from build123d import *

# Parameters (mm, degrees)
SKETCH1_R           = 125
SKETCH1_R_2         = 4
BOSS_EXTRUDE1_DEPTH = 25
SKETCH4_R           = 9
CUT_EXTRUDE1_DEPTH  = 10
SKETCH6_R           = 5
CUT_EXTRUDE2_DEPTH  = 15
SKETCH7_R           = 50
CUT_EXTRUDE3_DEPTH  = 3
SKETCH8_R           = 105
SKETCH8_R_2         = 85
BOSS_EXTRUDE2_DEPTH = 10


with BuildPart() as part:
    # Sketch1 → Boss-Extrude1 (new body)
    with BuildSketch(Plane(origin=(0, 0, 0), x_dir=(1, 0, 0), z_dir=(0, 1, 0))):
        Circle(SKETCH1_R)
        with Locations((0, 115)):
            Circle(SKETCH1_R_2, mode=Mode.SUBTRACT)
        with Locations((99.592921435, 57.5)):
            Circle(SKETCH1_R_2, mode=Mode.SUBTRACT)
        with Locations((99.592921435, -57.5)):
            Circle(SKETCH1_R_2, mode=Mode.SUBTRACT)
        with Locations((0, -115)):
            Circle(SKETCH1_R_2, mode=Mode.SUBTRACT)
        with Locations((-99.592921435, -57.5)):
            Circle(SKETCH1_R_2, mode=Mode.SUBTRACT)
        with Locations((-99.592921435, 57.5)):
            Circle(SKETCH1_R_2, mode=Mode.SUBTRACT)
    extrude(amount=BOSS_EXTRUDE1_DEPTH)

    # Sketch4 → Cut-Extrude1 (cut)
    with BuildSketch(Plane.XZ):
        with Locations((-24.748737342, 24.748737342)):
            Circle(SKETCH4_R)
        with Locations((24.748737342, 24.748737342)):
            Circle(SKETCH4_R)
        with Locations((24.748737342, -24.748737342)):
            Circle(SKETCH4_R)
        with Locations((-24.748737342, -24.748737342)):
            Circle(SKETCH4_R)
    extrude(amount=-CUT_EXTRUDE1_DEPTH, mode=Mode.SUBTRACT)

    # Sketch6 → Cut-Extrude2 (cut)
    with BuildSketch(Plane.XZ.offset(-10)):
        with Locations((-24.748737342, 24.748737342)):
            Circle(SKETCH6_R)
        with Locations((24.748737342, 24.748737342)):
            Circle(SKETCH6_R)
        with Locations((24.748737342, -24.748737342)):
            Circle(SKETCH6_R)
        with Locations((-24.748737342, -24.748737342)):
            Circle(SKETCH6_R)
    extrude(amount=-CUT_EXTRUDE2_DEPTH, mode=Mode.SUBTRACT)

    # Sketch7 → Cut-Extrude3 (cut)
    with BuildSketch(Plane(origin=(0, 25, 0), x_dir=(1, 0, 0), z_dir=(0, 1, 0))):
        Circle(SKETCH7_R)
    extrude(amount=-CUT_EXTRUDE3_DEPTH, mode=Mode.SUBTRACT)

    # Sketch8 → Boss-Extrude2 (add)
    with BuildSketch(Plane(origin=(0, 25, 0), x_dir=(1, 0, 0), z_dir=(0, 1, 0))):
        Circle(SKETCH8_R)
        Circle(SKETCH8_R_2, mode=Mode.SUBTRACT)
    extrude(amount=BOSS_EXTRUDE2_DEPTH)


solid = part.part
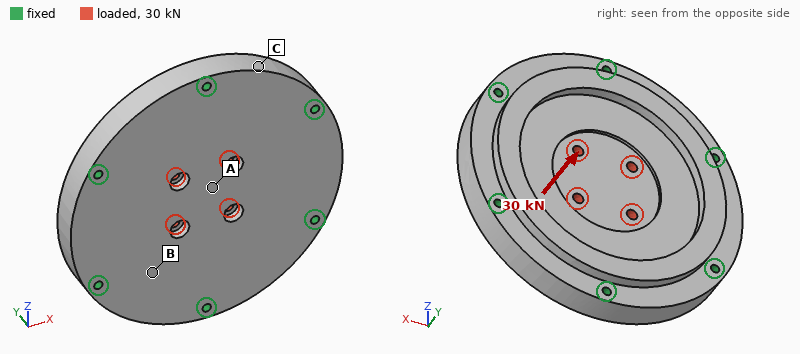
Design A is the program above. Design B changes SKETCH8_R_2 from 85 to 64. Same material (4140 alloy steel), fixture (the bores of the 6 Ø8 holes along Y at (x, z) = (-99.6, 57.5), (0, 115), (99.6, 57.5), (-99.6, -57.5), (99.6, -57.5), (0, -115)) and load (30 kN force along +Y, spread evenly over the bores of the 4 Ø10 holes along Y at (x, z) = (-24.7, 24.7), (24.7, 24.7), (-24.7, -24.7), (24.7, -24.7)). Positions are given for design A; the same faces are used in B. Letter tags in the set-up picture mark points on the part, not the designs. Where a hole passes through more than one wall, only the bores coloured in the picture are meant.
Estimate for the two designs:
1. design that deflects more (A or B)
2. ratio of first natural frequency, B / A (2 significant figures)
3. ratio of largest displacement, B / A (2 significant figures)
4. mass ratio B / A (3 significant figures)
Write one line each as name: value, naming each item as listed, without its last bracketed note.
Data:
design that deflects more: A
ratio of first natural frequency, B / A: 1.0
ratio of largest displacement, B / A: 0.85
mass ratio B / A: 1.08
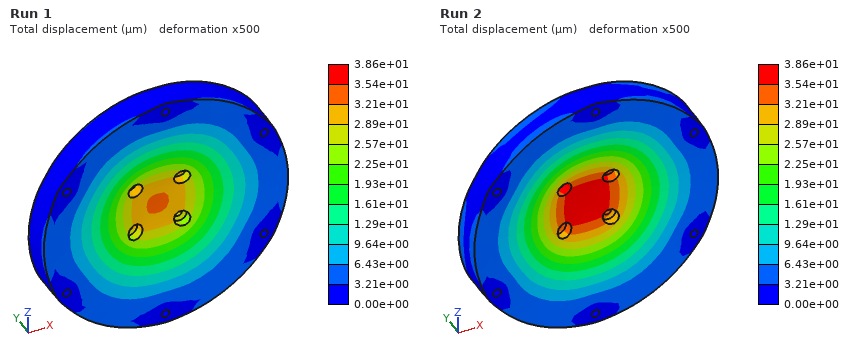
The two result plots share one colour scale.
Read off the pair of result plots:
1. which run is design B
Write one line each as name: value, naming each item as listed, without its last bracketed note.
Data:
which run is design B: Run 1
